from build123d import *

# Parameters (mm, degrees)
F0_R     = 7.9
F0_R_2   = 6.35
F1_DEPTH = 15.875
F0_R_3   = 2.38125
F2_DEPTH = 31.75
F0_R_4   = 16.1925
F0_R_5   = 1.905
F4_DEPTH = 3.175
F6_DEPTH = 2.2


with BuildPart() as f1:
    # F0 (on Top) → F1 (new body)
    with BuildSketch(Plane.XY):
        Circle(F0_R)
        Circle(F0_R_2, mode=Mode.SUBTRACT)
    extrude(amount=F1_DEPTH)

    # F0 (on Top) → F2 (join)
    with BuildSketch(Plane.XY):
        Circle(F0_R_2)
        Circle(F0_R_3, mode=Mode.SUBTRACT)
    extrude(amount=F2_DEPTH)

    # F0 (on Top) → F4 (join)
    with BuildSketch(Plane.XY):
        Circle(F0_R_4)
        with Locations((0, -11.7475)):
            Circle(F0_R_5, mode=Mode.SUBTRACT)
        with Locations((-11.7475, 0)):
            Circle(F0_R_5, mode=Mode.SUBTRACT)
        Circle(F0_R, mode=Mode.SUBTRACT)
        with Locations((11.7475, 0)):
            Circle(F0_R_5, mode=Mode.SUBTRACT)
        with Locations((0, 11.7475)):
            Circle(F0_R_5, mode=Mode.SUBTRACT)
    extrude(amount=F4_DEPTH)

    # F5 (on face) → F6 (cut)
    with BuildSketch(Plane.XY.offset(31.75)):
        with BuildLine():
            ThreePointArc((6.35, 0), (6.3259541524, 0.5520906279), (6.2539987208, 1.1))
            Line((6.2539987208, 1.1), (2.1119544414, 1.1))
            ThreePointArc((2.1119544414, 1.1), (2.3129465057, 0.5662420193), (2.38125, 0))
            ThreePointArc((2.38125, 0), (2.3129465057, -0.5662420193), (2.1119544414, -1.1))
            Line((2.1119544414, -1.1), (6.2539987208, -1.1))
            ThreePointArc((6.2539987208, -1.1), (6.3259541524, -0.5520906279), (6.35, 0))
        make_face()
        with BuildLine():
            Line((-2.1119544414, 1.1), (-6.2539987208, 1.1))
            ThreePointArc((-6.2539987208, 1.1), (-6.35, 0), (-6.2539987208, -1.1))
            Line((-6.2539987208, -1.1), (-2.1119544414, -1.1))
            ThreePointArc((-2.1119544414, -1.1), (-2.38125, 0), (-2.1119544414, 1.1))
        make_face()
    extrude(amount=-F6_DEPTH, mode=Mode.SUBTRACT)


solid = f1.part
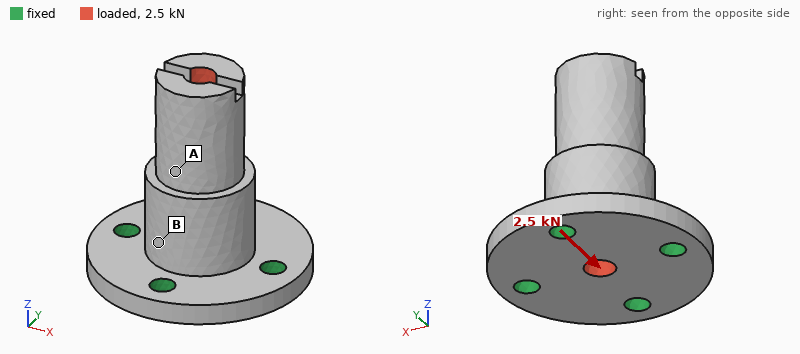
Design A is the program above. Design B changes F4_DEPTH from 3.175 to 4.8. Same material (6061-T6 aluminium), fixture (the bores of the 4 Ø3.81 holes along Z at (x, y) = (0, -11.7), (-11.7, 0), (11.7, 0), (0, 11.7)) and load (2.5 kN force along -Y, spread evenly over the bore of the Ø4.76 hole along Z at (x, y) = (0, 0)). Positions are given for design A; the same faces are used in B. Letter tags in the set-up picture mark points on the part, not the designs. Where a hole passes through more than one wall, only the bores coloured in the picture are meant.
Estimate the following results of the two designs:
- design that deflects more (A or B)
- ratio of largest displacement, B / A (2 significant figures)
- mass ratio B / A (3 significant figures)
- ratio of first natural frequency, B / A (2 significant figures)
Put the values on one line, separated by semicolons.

A; 0.66; 1.15; 1.2
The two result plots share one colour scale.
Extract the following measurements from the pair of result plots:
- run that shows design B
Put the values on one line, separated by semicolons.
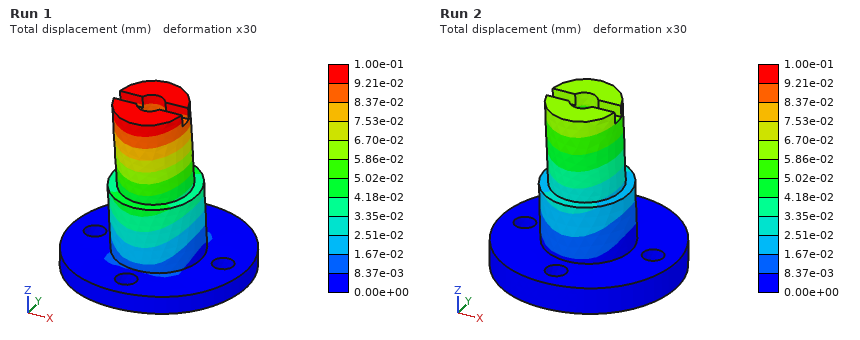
Run 2
